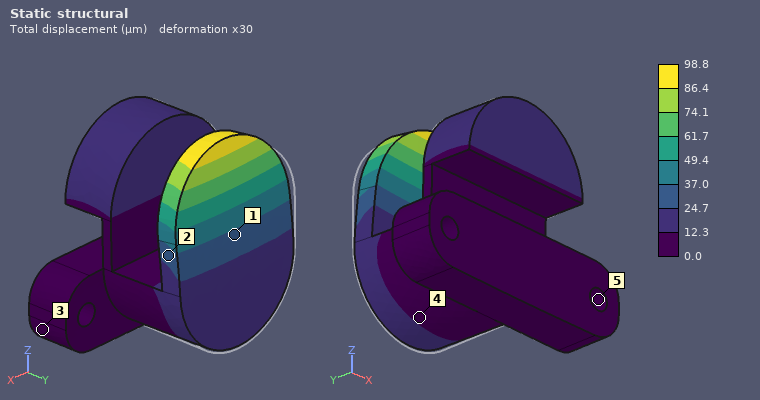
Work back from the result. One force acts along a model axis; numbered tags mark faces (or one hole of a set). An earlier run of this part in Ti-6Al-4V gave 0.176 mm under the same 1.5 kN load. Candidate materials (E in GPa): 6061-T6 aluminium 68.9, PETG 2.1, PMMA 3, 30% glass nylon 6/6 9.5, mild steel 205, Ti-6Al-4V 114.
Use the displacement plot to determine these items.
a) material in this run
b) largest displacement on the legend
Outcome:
mild steel
98.8 µm
